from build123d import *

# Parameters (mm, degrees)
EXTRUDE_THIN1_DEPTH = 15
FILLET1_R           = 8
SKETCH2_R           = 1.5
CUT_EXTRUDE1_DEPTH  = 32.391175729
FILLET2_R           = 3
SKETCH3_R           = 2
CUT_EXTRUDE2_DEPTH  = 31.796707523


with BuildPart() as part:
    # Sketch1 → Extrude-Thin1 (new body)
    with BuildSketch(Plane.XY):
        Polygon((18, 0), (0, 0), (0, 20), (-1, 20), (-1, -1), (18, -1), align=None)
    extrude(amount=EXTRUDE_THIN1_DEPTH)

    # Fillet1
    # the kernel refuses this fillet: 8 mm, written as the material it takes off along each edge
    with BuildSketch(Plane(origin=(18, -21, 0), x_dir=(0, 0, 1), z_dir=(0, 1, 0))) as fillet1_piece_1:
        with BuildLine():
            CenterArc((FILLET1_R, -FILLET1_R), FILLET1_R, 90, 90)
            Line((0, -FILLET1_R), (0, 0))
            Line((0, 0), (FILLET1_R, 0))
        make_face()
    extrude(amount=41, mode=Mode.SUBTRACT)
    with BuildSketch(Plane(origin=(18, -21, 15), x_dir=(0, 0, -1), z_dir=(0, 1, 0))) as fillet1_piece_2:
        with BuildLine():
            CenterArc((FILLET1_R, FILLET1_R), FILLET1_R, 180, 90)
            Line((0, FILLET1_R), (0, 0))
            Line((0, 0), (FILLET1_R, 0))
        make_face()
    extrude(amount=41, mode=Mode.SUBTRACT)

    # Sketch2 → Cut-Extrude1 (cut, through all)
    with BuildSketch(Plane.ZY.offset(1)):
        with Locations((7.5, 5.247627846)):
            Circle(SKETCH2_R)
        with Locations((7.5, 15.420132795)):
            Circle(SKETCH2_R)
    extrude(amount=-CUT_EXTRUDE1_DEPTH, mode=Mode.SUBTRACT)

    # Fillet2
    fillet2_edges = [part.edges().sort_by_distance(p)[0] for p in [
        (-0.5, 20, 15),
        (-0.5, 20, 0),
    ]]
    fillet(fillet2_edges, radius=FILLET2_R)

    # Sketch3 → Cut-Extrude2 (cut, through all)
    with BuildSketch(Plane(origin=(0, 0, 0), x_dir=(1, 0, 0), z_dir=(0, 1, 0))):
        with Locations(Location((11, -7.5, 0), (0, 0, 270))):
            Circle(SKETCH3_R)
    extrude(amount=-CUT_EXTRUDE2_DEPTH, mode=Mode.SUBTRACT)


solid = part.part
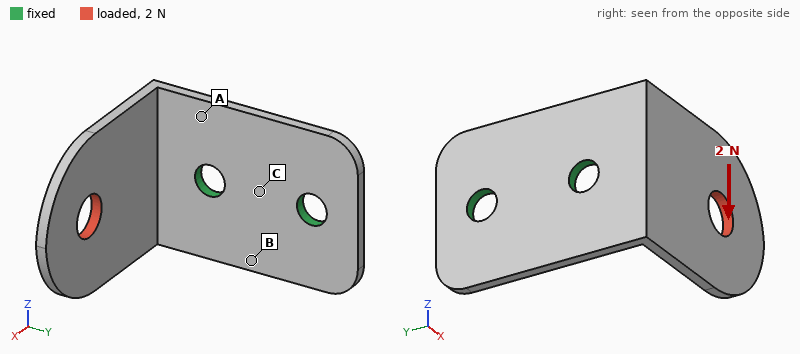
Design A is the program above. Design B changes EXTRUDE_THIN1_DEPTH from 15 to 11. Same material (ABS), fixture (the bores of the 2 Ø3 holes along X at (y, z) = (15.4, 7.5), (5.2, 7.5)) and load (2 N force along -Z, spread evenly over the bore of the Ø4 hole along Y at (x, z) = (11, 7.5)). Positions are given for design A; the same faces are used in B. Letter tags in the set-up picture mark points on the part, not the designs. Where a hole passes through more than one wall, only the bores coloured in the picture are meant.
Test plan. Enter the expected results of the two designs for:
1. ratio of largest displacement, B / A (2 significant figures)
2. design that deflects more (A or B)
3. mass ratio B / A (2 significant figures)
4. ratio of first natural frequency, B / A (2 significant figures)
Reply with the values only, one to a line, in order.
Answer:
1.4
B
0.73
0.97
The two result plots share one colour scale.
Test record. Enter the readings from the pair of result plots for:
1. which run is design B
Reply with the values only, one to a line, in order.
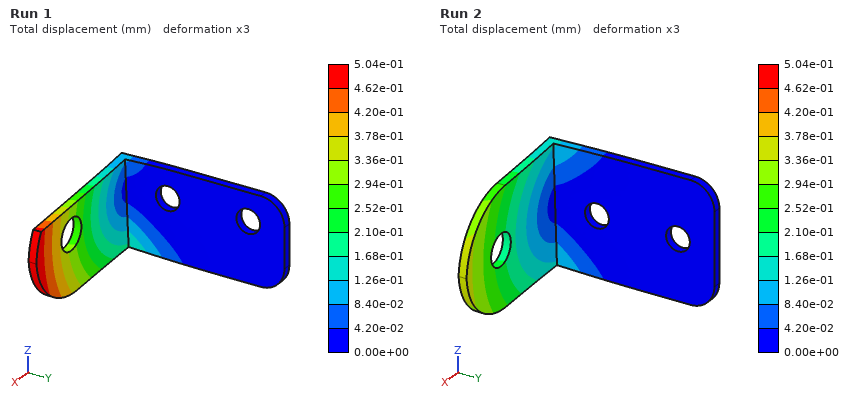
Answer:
Run 1
